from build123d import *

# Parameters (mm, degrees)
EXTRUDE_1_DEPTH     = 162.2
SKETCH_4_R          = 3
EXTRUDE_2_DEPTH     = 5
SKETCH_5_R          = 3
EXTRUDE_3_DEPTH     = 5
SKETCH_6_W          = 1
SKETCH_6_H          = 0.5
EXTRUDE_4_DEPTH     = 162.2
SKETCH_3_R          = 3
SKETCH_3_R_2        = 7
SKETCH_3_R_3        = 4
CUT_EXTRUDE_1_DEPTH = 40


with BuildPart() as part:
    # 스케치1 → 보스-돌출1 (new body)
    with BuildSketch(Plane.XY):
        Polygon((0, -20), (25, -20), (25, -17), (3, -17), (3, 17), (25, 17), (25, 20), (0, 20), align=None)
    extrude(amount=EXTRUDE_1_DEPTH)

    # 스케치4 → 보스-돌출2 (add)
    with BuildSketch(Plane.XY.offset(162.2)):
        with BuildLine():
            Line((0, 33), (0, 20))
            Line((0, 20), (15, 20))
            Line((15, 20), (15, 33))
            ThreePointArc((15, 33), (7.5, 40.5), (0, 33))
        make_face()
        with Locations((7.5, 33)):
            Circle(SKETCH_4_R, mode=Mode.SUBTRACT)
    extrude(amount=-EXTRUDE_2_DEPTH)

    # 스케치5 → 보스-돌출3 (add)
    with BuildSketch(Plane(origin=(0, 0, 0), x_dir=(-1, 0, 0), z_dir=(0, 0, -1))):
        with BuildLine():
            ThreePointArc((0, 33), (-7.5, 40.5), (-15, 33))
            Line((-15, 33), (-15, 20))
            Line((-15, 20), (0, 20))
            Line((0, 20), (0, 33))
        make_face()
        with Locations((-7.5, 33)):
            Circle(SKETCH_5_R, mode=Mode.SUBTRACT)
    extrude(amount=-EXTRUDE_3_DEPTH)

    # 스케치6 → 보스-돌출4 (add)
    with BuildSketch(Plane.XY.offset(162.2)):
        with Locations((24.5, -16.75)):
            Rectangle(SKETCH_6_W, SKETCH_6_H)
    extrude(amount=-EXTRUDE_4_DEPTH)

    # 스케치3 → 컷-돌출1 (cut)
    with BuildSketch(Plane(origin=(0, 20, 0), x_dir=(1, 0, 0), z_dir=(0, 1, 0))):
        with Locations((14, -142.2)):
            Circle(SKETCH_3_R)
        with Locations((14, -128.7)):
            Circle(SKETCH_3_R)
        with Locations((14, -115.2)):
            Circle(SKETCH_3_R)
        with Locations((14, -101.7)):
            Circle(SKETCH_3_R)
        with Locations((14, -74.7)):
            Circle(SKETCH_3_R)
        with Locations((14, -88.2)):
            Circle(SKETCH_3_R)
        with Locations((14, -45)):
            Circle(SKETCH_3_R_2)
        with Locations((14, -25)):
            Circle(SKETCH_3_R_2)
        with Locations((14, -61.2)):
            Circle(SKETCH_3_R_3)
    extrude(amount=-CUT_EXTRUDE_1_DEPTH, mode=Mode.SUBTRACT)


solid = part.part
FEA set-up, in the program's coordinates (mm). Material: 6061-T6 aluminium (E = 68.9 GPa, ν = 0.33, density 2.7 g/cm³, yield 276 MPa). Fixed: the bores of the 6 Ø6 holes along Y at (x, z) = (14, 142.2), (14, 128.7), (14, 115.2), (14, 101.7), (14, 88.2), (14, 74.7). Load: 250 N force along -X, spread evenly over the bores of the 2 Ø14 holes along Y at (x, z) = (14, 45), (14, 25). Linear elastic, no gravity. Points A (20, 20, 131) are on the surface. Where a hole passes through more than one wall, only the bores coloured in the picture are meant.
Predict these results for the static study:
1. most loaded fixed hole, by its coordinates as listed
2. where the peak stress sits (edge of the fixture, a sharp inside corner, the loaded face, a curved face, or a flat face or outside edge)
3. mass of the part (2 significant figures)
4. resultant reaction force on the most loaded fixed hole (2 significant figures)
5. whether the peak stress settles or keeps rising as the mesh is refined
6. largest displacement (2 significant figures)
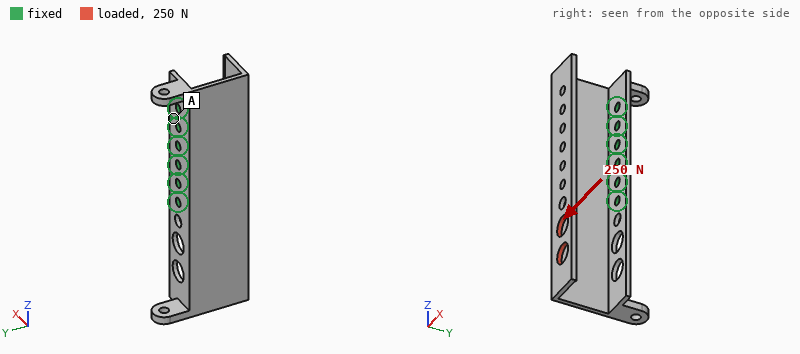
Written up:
(14, 74.7)
edge of the fixture
110 g
460 N
keeps rising
1.3 mm
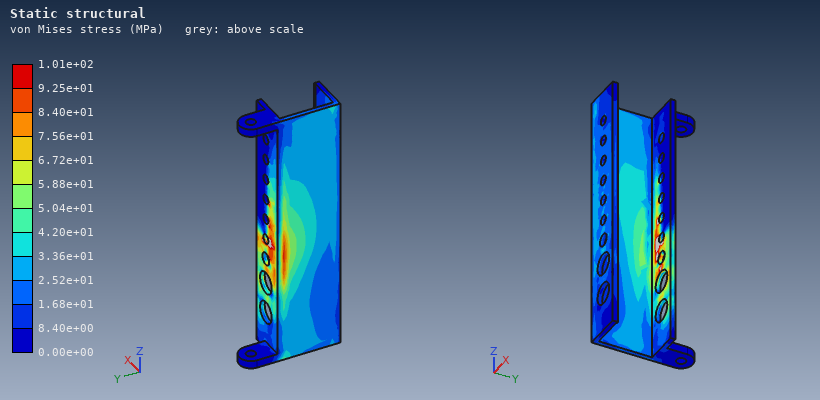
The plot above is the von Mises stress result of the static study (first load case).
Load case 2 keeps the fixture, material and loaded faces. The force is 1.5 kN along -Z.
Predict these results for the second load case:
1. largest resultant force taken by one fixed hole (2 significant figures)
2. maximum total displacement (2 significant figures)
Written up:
700 N
1.2 mm
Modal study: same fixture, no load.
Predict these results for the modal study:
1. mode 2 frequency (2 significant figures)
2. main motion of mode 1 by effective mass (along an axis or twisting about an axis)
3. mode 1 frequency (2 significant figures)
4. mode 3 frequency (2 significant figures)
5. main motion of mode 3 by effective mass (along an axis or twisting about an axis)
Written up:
840 Hz
along X
530 Hz
1300 Hz
along Y
